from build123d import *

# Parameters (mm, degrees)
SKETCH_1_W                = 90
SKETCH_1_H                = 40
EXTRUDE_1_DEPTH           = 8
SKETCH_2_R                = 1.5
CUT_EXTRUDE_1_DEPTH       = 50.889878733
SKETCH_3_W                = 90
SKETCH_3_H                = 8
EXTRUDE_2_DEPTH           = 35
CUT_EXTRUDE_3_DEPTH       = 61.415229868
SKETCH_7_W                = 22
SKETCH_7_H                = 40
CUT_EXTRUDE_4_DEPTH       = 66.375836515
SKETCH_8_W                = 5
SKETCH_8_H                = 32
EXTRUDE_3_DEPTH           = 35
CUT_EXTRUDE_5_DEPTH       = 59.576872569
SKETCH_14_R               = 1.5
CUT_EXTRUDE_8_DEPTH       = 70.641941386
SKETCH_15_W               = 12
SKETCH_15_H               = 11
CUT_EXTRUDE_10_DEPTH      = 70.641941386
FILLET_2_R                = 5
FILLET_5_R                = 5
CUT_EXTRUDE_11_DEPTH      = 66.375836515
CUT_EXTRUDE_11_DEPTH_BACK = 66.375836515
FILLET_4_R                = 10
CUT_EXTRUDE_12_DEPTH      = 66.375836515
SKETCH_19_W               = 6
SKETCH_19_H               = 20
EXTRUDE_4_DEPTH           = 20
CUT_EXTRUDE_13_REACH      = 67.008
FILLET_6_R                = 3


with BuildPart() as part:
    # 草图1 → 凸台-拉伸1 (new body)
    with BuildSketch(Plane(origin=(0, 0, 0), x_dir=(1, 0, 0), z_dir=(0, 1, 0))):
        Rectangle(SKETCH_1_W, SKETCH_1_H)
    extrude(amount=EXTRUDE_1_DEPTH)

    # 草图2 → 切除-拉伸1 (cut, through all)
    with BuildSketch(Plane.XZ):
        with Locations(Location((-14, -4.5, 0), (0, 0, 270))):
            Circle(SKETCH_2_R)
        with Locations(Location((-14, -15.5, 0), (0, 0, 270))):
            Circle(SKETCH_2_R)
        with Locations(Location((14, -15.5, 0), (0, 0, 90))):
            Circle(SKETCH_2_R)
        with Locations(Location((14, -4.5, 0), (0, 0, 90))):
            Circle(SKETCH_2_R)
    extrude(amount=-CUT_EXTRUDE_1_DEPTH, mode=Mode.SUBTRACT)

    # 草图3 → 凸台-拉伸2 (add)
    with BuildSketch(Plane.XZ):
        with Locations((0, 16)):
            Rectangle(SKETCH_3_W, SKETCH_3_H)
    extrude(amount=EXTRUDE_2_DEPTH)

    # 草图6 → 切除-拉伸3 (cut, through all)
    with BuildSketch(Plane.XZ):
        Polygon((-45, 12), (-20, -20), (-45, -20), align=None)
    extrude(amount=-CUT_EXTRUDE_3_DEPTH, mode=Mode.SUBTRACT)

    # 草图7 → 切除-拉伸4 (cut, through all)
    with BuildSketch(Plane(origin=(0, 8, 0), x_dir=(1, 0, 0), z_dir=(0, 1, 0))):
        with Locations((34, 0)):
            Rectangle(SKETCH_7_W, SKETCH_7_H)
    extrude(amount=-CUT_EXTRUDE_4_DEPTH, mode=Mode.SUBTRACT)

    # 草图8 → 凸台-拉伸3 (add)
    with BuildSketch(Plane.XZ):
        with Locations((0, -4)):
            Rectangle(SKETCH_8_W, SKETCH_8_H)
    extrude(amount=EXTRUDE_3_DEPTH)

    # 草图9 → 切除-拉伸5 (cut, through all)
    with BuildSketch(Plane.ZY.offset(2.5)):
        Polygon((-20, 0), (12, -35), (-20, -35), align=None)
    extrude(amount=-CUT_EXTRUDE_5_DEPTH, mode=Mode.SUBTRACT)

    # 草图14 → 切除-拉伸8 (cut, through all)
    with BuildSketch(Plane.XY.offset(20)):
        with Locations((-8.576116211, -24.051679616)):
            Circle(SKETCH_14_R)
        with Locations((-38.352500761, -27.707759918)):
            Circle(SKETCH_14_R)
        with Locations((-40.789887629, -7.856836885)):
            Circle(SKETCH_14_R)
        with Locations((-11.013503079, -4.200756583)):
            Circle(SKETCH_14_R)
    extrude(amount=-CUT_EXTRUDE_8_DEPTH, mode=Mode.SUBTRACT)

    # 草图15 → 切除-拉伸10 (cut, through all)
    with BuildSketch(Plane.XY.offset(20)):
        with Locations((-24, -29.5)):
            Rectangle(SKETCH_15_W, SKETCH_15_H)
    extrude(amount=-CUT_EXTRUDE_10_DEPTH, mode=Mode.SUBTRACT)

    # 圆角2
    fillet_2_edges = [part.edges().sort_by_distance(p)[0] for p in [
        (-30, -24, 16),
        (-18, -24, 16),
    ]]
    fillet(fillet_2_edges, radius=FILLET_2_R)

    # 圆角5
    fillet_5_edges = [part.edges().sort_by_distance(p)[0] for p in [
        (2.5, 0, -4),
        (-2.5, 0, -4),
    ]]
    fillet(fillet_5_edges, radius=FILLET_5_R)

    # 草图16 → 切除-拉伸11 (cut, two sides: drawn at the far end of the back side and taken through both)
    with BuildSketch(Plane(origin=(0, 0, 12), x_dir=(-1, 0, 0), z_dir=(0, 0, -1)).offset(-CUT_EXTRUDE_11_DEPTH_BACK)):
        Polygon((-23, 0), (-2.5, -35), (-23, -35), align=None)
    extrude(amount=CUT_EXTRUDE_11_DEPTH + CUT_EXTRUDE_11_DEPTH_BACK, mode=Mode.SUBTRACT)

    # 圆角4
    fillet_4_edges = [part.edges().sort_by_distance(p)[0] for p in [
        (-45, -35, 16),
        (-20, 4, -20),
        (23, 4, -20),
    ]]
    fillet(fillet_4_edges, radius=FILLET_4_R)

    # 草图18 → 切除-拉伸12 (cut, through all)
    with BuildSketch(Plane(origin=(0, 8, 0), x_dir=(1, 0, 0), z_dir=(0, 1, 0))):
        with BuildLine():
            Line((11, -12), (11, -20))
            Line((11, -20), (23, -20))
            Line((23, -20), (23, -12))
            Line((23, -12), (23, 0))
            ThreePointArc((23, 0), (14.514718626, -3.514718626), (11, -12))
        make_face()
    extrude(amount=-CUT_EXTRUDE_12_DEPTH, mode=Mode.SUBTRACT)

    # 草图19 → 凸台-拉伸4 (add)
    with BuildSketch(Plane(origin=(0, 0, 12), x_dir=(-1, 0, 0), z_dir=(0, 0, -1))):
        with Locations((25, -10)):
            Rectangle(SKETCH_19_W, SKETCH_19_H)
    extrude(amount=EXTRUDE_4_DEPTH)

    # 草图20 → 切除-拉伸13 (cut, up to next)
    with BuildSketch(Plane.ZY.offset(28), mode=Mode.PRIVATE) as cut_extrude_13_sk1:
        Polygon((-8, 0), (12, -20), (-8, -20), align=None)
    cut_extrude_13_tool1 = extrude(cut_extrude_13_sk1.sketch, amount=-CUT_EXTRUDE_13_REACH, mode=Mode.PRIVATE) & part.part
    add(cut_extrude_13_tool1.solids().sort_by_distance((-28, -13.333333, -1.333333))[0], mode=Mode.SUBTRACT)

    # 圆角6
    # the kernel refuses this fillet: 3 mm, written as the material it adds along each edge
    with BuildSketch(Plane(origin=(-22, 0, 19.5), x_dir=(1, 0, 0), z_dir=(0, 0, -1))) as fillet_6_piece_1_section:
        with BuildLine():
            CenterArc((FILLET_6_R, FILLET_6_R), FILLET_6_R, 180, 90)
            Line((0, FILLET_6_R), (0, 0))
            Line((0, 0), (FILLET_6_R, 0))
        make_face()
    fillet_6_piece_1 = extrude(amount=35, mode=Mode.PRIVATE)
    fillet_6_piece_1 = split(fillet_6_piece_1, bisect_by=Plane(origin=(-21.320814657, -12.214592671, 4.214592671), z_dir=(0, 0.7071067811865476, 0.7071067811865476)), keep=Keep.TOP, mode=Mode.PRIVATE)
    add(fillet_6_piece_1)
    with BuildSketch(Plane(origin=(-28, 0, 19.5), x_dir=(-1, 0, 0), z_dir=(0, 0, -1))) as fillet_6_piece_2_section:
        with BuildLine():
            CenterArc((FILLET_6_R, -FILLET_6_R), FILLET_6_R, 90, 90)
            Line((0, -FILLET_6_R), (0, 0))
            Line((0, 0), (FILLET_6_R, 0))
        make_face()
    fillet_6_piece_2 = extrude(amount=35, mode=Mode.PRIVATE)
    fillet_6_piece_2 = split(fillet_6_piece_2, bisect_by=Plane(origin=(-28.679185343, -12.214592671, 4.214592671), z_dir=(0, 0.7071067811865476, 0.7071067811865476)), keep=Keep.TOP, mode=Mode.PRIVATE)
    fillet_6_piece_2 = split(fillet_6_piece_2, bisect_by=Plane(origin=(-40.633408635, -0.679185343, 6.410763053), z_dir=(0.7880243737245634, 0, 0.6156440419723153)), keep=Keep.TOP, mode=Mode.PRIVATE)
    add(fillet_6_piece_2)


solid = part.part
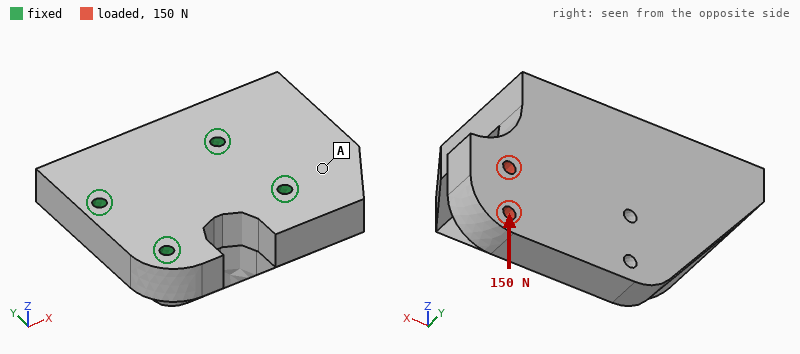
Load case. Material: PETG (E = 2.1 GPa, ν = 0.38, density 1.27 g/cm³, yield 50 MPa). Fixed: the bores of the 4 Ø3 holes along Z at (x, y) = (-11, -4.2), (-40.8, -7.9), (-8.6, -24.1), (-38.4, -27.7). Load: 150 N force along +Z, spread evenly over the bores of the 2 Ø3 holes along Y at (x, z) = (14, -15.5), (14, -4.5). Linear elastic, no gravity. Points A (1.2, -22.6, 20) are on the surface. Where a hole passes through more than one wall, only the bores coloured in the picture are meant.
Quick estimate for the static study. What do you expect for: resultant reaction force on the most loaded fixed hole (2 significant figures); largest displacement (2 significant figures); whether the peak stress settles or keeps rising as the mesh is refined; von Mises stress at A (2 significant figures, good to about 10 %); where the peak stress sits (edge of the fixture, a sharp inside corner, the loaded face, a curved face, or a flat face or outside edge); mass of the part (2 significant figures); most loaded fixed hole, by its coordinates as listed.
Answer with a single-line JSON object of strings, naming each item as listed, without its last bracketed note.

{"resultant reaction force on the most loaded fixed hole": "260 N", "largest displacement": "0.20 mm", "whether the peak stress settles or keeps rising as the mesh is refined": "keeps rising", "von Mises stress at A": "0.99 MPa", "where the peak stress sits": "edge of the fixture", "mass of the part": "44 g", "most loaded fixed hole, by its coordinates as listed": "(-11, -4.2)"}
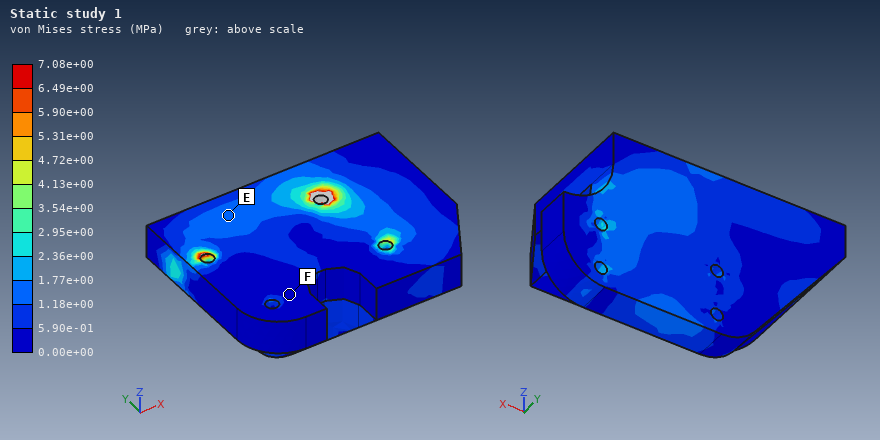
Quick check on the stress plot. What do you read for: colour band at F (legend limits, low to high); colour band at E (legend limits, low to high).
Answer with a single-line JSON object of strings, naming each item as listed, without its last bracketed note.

{"colour band at F": "0.00e+00 to 5.90e-01 MPa", "colour band at E": "1.18e+00 to 1.77e+00 MPa"}
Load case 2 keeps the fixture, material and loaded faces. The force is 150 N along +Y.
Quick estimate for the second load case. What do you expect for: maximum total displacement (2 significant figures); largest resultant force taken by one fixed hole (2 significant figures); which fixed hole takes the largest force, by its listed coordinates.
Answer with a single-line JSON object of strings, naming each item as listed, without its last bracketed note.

{"maximum total displacement": "0.36 mm", "largest resultant force taken by one fixed hole": "230 N", "which fixed hole takes the largest force, by its listed coordinates": "(-8.6, -24.1)"}
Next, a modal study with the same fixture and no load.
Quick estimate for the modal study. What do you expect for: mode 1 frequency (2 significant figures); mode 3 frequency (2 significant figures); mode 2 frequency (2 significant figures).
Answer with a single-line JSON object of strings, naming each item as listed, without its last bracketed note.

{"mode 1 frequency": "1400 Hz", "mode 3 frequency": "2500 Hz", "mode 2 frequency": "2000 Hz"}
